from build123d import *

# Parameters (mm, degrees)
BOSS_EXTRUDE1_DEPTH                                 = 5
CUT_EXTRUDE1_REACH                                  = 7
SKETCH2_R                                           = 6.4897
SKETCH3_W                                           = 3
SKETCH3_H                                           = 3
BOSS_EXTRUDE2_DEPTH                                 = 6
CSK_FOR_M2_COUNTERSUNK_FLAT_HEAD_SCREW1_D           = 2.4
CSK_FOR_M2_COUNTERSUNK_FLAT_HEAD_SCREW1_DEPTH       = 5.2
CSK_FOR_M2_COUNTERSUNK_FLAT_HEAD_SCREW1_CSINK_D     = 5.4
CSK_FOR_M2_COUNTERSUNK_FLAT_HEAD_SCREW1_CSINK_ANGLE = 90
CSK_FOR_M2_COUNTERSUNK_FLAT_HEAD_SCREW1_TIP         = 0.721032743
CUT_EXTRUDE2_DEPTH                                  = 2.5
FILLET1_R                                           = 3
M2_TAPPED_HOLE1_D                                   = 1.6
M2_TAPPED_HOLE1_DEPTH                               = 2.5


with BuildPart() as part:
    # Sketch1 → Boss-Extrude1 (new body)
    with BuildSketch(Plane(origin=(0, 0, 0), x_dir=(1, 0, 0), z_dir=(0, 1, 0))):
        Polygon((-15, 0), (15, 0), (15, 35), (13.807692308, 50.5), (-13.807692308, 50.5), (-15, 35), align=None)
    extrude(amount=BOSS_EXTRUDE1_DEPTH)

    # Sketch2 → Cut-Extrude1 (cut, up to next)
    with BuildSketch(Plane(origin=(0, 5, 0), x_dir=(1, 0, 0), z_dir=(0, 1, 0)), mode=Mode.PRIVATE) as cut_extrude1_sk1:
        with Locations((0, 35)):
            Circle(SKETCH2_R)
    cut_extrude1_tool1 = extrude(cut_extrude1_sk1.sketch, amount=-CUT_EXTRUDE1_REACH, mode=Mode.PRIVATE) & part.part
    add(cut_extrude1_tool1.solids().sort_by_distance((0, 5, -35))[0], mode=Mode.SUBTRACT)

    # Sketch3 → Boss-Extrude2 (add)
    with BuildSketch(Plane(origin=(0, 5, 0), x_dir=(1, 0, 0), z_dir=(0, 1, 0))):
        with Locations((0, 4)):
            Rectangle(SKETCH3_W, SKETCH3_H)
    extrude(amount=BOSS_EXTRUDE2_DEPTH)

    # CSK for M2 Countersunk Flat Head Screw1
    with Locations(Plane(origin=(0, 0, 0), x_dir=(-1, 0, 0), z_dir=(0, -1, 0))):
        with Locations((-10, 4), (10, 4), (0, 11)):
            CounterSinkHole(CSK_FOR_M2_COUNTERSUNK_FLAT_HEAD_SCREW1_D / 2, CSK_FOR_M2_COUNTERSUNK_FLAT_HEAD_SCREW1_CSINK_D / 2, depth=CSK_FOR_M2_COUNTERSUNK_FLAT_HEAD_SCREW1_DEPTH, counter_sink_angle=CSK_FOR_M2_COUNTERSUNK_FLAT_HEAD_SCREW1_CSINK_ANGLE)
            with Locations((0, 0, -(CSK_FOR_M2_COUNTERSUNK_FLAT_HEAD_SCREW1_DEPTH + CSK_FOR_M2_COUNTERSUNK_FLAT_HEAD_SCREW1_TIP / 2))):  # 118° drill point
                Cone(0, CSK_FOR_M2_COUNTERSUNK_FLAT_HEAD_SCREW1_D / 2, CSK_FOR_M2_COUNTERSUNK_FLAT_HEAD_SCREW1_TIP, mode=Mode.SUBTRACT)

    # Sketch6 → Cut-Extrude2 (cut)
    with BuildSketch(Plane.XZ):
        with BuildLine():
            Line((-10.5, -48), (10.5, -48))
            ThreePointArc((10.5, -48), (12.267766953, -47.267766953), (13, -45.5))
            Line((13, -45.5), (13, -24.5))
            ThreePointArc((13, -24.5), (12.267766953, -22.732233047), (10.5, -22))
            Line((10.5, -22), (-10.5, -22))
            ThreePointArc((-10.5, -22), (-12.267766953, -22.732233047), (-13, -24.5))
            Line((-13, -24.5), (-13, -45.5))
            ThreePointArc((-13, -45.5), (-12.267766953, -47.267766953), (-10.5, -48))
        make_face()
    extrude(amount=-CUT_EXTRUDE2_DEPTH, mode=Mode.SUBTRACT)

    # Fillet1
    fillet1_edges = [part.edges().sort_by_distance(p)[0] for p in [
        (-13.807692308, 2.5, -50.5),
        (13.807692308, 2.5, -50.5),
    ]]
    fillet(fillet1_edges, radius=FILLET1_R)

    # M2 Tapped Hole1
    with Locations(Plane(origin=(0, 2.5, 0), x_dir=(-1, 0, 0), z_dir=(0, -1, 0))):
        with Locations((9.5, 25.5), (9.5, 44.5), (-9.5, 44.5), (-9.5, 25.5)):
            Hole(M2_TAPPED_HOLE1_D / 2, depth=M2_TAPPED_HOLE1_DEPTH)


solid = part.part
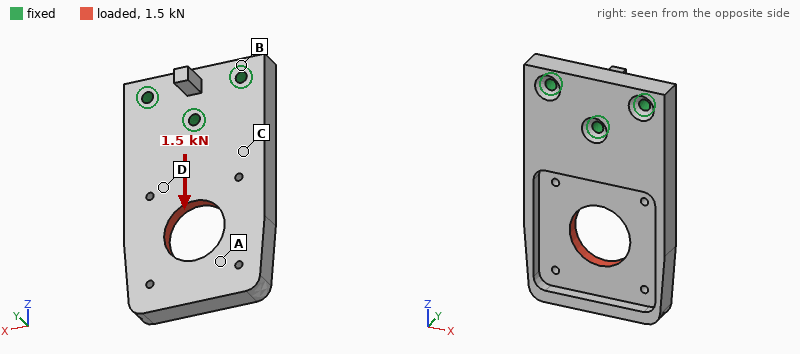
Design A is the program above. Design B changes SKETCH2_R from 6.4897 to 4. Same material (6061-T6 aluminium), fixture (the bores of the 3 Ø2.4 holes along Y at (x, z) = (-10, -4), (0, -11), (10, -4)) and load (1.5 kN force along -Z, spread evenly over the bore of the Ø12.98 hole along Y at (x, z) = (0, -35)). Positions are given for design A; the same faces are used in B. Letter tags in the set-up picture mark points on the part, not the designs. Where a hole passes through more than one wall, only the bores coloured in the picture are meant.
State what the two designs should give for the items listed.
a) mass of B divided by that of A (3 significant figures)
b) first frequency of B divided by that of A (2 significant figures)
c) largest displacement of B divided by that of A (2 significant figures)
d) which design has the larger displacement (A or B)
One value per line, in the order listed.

1.04
1.00
0.89
A
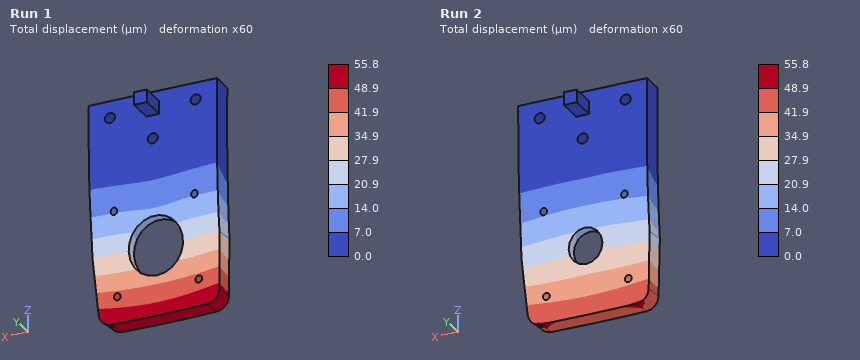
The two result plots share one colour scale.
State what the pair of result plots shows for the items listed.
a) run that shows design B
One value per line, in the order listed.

Run 2
